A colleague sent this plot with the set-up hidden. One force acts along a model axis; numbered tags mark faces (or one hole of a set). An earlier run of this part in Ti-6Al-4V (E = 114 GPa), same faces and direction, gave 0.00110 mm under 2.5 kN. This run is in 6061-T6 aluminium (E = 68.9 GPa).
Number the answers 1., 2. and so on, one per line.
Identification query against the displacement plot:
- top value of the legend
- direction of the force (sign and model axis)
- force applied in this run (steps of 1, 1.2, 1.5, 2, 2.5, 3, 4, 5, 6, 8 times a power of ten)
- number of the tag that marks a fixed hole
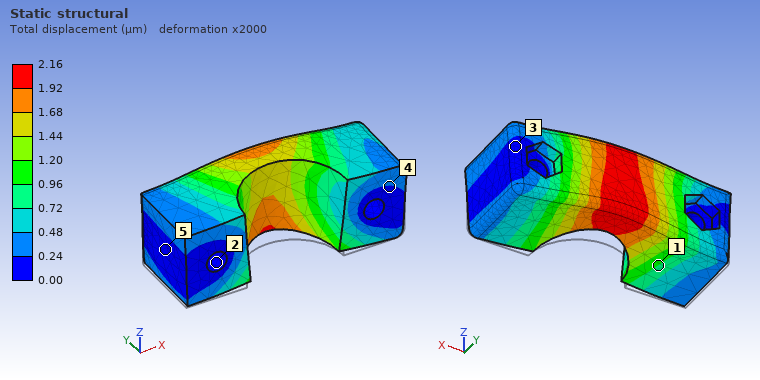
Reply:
1. 2.16 µm
2. +Z
3. 3 kN
4. 2
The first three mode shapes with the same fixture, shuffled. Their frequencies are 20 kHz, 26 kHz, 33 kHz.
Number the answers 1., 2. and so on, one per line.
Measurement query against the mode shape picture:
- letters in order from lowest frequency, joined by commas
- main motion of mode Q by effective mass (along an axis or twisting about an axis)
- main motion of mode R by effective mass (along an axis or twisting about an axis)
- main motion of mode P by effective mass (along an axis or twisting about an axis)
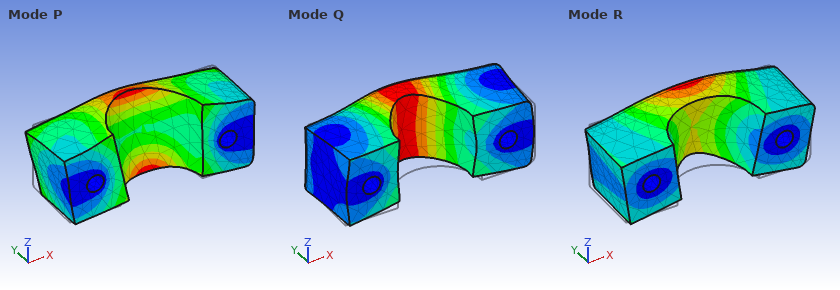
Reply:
1. R, Q, P
2. along Y
3. along Z
4. twisting about X
